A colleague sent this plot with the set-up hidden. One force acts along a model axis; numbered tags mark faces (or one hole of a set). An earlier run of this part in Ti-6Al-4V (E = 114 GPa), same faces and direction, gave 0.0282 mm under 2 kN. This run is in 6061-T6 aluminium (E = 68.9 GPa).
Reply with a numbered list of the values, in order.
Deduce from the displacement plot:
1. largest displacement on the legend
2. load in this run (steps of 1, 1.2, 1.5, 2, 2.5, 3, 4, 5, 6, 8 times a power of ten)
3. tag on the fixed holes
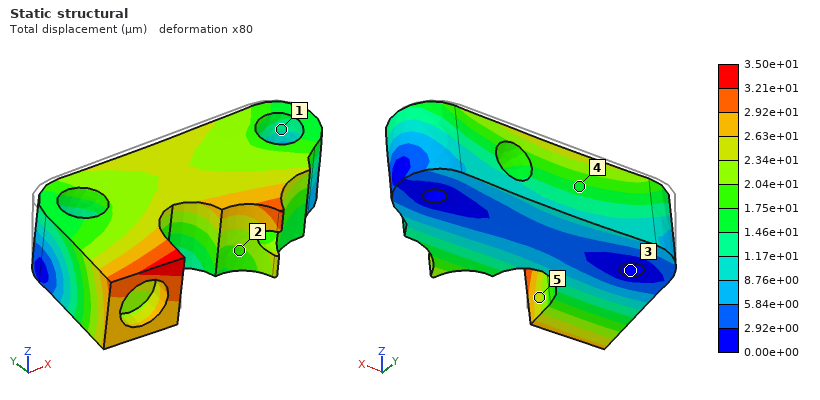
1. 3.50e+01 µm
2. 1.5 kN
3. 3
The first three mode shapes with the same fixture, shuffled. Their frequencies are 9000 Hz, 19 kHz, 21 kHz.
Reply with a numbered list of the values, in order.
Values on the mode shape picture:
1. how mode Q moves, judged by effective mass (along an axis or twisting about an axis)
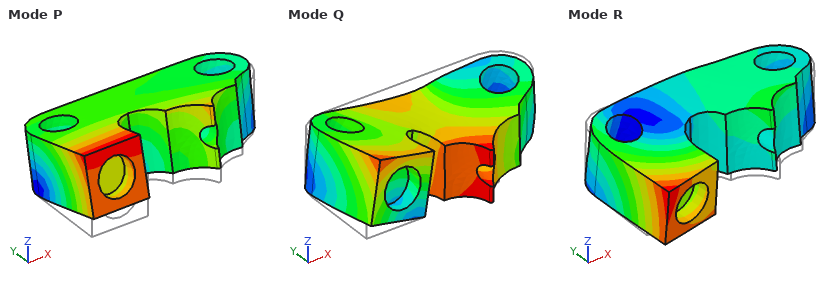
1. along Z
